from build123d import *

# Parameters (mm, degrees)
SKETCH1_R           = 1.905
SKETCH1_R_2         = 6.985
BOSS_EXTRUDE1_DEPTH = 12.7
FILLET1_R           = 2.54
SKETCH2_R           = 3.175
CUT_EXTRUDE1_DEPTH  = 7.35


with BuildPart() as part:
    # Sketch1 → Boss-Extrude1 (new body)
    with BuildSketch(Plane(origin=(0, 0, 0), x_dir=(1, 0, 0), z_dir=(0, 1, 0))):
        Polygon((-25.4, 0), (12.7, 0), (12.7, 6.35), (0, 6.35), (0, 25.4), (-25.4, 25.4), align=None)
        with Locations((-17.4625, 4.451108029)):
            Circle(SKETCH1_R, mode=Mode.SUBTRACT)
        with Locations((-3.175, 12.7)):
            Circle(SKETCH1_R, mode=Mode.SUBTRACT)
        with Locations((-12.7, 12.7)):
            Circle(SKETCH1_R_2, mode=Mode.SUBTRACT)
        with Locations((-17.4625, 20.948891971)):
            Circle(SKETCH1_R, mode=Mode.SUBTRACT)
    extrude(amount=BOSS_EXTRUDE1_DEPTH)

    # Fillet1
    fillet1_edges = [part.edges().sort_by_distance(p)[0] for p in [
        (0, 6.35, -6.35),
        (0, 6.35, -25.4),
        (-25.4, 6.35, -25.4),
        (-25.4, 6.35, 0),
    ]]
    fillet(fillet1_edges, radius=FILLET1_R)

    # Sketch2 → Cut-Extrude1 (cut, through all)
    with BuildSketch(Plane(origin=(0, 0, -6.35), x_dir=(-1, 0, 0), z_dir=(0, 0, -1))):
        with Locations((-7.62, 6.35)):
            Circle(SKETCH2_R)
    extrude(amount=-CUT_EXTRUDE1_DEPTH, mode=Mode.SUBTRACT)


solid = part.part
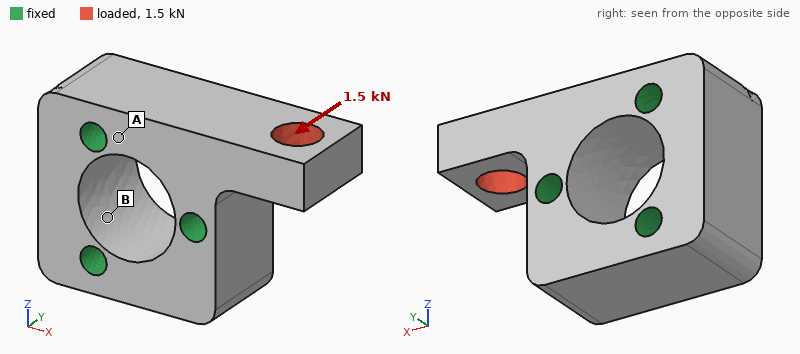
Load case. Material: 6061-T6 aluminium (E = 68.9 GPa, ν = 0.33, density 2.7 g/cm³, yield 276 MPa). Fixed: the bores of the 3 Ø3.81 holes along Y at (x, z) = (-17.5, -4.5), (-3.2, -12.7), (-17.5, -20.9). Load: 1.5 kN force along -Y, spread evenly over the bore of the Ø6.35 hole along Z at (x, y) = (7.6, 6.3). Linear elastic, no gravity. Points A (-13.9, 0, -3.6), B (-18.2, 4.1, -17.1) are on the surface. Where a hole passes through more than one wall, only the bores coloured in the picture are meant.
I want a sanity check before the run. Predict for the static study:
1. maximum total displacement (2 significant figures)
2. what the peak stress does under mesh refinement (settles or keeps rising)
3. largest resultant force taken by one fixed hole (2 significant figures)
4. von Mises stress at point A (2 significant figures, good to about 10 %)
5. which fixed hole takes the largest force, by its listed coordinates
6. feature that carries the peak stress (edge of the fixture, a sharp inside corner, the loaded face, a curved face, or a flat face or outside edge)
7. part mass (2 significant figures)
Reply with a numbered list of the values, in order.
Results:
1. 65 µm
2. keeps rising
3. 1.7 kN
4. 49 MPa
5. (-3.2, -12.7)
6. edge of the fixture
7. 18 g
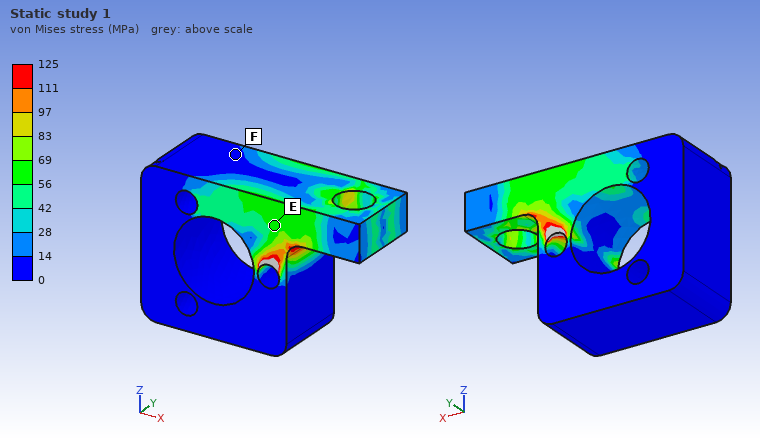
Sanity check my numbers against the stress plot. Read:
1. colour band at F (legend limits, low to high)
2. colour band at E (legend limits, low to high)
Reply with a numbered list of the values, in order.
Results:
1. 0 to 14 MPa
2. 56 to 69 MPa
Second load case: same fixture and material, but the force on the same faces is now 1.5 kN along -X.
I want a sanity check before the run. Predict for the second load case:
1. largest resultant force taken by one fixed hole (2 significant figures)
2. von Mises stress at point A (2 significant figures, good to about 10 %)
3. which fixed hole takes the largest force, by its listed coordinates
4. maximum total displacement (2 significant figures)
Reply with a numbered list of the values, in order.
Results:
1. 1.1 kN
2. 18 MPa
3. (-17.5, -4.5)
4. 14 µm
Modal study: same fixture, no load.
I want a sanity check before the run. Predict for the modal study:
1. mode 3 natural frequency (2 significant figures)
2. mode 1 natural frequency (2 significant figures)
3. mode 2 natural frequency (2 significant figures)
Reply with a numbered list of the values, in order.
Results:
1. 35 kHz
2. 20 kHz
3. 21 kHz
